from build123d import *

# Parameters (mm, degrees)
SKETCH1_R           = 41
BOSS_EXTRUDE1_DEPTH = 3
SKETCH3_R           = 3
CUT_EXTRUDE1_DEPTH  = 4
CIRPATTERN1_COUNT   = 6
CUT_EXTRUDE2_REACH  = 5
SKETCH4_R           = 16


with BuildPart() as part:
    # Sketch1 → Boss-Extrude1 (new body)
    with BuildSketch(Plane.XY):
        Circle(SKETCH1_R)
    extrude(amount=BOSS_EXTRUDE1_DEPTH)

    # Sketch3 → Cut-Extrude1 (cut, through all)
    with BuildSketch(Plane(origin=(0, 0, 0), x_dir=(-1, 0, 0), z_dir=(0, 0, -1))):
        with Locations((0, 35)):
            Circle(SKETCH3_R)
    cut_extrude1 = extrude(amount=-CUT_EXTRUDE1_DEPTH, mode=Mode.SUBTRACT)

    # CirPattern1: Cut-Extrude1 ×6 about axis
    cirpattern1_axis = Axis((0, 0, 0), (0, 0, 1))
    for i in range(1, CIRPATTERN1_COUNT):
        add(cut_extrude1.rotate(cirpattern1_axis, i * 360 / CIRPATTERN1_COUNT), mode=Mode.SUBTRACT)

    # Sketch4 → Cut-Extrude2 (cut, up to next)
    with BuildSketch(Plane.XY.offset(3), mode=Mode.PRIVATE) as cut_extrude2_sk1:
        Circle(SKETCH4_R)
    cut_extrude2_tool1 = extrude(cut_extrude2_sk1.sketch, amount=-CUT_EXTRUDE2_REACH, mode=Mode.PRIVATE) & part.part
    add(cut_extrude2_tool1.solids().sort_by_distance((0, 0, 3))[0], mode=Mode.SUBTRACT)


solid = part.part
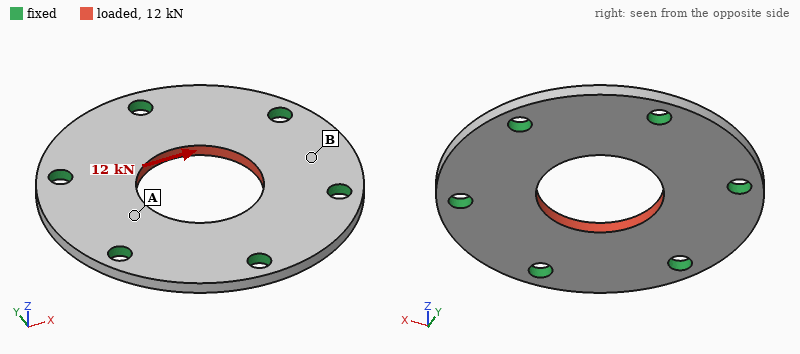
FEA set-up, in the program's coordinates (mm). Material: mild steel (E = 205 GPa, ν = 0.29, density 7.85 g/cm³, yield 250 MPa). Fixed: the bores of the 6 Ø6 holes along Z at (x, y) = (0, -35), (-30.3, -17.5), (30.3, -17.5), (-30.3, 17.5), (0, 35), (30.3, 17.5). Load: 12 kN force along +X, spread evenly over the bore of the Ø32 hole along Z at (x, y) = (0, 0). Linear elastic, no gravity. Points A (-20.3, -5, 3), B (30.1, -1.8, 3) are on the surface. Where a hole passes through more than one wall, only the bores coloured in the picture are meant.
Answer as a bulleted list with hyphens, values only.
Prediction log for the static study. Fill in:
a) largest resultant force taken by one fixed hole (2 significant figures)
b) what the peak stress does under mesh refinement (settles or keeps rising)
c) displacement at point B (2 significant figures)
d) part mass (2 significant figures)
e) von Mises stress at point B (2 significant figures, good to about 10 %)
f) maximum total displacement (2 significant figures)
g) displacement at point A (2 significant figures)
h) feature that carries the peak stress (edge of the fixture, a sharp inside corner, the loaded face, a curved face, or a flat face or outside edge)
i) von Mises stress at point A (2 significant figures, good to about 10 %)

- 2.5 kN
- keeps rising
- 3.5 µm
- 100 g
- 13 MPa
- 5.3 µm
- 4.2 µm
- edge of the fixture
- 35 MPa
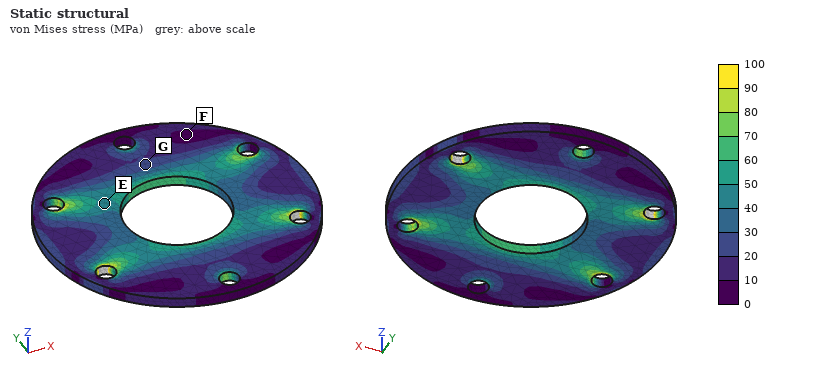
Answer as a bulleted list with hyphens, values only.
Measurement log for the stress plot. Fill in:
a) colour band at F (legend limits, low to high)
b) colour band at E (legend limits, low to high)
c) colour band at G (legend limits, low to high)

- 0 to 10 MPa
- 40 to 50 MPa
- 20 to 30 MPa
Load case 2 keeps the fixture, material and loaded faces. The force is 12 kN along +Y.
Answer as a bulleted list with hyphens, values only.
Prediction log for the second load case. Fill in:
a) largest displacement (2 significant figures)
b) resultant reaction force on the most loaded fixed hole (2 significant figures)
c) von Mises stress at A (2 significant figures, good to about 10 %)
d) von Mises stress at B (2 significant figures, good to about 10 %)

- 5.3 µm
- 2.8 kN
- 44 MPa
- 14 MPa
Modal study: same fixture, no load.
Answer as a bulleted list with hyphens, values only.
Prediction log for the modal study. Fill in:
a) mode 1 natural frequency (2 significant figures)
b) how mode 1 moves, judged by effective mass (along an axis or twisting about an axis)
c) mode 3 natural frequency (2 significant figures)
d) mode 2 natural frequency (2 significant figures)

- 8500 Hz
- along Z
- 11 kHz
- 11 kHz
